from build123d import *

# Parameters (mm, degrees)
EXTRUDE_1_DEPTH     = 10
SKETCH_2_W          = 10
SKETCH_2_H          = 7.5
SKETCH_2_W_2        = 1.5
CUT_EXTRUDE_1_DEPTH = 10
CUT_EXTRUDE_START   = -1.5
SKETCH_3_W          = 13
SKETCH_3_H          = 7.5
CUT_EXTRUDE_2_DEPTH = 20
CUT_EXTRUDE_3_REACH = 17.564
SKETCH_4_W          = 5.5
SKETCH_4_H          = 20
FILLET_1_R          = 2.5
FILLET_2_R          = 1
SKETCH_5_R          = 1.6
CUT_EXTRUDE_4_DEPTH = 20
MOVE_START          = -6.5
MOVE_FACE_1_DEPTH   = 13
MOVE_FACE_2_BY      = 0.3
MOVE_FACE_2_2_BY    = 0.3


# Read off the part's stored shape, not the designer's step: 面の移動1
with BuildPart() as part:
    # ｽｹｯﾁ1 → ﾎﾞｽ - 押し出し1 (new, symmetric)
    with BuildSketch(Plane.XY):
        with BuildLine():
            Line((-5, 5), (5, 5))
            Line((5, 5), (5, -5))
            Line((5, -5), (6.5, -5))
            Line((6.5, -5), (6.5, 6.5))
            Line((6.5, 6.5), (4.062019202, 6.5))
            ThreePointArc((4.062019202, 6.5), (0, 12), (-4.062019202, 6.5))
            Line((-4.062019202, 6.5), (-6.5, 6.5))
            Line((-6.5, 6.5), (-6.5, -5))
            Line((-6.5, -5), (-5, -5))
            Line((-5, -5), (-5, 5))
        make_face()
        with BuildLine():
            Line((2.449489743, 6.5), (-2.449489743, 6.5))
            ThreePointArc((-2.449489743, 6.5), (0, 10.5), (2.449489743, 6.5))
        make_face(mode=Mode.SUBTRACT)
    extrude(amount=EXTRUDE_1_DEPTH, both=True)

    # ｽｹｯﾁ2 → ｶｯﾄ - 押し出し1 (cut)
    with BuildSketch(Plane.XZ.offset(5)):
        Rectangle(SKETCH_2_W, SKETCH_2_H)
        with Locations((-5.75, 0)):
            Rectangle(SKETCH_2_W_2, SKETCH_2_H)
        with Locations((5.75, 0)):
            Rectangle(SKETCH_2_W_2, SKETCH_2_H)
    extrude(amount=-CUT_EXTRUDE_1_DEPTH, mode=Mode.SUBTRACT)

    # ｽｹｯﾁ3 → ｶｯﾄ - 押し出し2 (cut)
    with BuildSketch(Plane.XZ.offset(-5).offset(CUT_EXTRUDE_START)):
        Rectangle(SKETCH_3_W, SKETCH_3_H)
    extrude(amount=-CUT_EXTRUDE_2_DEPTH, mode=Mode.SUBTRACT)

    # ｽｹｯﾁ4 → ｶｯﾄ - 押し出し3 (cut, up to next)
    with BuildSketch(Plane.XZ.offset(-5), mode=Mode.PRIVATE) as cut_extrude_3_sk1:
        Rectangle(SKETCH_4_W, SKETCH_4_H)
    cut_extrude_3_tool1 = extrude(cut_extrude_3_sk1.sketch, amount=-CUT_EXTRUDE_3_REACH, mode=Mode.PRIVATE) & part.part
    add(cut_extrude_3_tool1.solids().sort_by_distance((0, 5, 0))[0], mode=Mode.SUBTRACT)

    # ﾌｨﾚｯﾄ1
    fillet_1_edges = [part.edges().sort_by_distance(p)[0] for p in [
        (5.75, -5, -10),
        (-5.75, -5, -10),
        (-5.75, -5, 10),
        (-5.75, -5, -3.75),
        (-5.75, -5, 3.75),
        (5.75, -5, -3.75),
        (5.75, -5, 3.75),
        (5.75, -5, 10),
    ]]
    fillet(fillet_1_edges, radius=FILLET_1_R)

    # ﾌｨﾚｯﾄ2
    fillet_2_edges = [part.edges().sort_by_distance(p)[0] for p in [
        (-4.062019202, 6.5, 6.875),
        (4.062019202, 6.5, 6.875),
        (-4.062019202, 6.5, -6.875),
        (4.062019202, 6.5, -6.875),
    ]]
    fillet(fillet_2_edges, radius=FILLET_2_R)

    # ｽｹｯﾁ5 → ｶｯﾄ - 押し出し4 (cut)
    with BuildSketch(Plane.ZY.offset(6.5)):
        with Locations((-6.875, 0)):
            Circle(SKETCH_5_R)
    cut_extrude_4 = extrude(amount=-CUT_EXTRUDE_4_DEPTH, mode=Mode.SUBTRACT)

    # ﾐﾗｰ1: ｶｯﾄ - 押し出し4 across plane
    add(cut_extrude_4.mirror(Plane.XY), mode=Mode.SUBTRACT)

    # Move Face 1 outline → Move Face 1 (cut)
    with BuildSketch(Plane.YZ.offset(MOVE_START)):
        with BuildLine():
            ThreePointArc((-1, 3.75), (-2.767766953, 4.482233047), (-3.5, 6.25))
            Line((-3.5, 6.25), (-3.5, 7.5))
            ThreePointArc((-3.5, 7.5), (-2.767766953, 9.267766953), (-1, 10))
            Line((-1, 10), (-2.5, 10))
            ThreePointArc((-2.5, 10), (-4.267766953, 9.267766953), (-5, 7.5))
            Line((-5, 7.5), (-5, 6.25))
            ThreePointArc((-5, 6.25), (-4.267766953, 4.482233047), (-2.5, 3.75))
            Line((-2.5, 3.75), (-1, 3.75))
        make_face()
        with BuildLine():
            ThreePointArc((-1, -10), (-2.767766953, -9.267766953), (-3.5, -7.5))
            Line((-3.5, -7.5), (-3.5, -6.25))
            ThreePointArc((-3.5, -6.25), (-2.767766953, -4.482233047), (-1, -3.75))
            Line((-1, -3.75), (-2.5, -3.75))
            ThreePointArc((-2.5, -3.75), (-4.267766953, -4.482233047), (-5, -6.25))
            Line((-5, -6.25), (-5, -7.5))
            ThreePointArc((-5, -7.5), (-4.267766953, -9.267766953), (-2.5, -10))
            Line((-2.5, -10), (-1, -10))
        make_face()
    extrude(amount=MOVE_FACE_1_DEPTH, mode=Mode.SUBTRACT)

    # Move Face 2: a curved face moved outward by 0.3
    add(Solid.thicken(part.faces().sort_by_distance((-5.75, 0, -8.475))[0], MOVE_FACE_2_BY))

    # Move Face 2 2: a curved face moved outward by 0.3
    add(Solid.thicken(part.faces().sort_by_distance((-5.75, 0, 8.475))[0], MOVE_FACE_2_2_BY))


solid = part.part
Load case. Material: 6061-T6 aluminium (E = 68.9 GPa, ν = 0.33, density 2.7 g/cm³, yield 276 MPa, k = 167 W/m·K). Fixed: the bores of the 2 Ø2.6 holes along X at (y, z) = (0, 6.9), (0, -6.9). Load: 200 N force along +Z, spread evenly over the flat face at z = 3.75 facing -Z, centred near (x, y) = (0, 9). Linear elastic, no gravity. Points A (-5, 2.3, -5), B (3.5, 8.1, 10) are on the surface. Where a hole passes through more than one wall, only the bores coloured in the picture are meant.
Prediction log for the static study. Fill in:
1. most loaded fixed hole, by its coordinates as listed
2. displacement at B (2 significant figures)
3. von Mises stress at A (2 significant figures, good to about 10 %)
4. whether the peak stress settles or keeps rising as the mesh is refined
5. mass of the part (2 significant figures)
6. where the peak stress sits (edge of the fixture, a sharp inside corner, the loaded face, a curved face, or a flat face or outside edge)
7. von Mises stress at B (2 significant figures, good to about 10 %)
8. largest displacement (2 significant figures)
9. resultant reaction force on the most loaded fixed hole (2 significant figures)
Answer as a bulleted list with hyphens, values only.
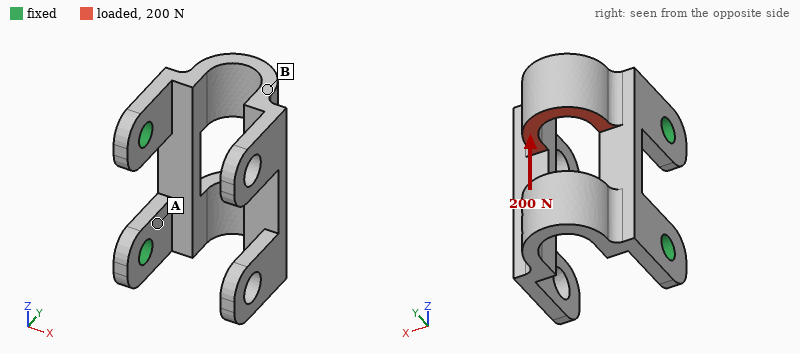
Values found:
- (0, -6.9)
- 0.10 mm
- 72 MPa
- keeps rising
- 2.0 g
- edge of the fixture
- 34 MPa
- 0.16 mm
- 160 N
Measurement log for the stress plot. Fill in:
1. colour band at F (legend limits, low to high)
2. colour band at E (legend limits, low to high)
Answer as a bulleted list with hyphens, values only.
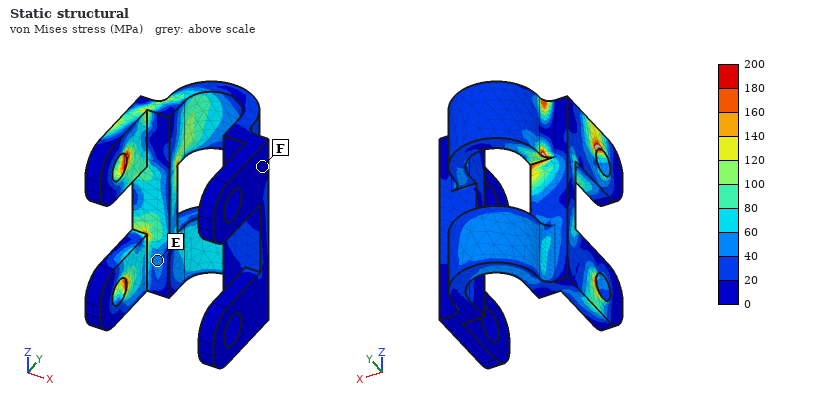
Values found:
- 0 to 20 MPa
- 40 to 60 MPa
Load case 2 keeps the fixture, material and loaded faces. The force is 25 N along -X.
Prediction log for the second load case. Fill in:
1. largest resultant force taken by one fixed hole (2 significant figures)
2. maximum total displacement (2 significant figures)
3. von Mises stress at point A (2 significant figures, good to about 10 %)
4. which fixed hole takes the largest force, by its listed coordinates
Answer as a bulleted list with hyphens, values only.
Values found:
- 18 N
- 54 µm
- 28 MPa
- (0, 6.9)
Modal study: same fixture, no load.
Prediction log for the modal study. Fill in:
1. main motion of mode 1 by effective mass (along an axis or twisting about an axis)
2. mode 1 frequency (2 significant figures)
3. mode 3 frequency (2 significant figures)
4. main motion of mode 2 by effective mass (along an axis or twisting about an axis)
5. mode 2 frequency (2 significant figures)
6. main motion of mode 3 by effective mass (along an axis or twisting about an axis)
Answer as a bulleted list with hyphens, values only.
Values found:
- along Y
- 2200 Hz
- 4300 Hz
- along Z
- 3500 Hz
- along X
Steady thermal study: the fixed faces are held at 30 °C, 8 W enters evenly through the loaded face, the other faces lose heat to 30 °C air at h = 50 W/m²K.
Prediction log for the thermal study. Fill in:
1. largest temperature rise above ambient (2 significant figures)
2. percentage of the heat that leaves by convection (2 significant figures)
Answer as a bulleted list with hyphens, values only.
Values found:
- 42 K
- 15 %
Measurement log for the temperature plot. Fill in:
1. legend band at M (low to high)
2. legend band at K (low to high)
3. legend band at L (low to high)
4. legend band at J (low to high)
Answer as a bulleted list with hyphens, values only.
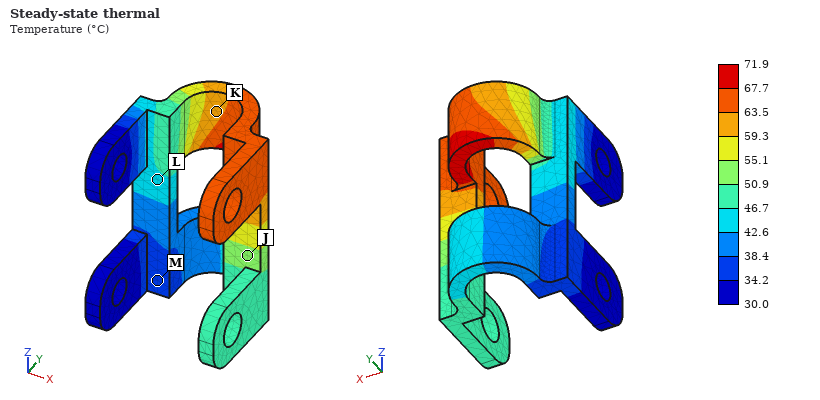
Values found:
- 34.2 to 38.4 °C
- 59.3 to 63.5 °C
- 42.6 to 46.7 °C
- 50.9 to 55.1 °C
